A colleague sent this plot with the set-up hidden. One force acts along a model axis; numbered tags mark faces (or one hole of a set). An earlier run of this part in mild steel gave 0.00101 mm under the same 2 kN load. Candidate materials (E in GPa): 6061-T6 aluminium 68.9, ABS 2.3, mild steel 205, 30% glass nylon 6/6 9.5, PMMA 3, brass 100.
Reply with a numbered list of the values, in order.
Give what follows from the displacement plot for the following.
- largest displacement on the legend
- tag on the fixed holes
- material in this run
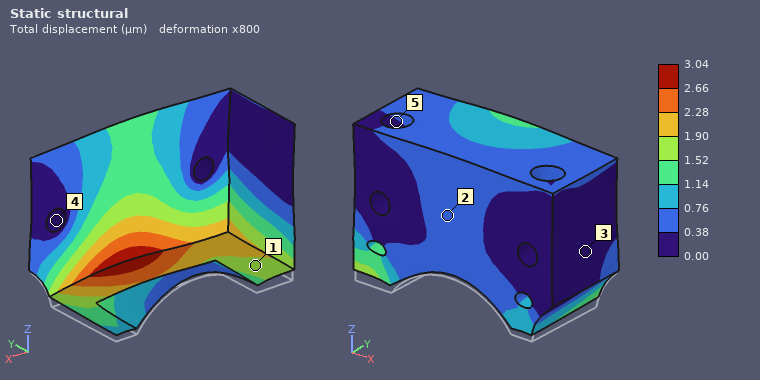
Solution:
1. 3.04 µm
2. 4
3. 6061-T6 aluminium
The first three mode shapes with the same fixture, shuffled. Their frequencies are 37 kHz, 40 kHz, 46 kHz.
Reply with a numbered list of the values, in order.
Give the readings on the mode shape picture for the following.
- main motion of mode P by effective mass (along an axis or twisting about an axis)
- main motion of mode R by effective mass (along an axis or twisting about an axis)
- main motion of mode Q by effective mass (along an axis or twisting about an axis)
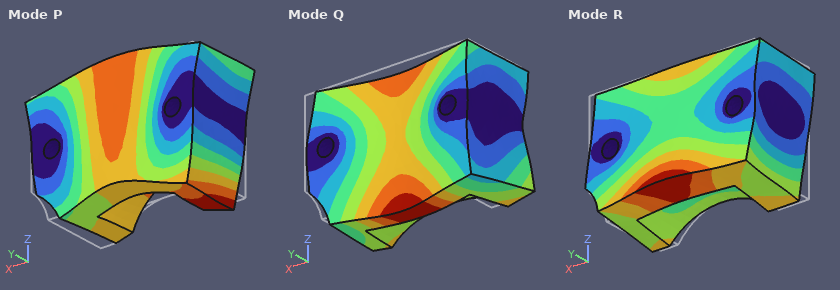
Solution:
1. along Z
2. twisting about X
3. along Y
